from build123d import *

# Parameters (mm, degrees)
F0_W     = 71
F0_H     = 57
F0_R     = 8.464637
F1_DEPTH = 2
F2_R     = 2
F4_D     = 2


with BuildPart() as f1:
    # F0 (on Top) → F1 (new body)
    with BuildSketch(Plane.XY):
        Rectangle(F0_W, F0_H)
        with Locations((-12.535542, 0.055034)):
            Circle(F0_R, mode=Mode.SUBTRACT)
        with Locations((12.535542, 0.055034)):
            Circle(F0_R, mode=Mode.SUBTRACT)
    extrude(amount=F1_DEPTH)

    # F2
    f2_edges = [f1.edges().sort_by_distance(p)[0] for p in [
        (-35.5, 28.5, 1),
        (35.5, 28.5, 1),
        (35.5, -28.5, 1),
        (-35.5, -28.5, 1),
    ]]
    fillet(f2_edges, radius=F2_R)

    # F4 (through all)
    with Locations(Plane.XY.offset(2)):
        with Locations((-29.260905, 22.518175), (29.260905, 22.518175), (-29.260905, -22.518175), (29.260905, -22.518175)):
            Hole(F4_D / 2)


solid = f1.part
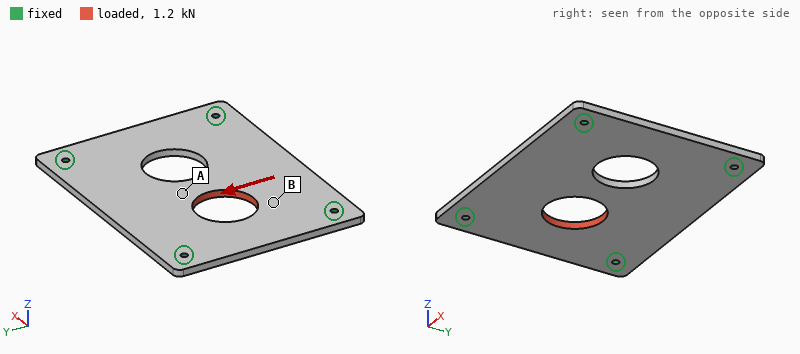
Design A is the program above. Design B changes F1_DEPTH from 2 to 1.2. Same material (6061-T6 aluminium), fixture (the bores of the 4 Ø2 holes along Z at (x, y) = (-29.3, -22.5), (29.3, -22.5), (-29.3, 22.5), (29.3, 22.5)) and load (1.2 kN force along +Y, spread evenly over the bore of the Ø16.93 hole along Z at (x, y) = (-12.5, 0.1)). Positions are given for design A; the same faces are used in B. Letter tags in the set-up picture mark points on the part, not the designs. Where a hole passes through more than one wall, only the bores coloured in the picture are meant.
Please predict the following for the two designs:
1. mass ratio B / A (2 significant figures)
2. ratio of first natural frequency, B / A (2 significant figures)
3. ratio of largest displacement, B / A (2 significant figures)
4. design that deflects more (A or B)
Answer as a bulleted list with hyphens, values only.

- 0.60
- 0.62
- 1.7
- B
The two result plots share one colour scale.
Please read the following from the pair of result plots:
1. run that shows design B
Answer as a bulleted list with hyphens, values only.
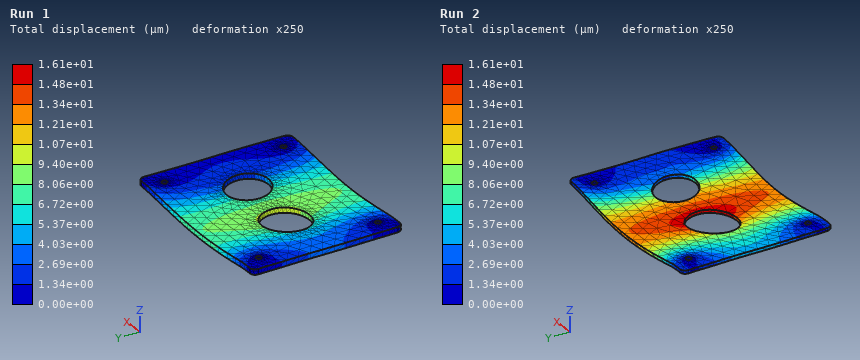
- Run 2
